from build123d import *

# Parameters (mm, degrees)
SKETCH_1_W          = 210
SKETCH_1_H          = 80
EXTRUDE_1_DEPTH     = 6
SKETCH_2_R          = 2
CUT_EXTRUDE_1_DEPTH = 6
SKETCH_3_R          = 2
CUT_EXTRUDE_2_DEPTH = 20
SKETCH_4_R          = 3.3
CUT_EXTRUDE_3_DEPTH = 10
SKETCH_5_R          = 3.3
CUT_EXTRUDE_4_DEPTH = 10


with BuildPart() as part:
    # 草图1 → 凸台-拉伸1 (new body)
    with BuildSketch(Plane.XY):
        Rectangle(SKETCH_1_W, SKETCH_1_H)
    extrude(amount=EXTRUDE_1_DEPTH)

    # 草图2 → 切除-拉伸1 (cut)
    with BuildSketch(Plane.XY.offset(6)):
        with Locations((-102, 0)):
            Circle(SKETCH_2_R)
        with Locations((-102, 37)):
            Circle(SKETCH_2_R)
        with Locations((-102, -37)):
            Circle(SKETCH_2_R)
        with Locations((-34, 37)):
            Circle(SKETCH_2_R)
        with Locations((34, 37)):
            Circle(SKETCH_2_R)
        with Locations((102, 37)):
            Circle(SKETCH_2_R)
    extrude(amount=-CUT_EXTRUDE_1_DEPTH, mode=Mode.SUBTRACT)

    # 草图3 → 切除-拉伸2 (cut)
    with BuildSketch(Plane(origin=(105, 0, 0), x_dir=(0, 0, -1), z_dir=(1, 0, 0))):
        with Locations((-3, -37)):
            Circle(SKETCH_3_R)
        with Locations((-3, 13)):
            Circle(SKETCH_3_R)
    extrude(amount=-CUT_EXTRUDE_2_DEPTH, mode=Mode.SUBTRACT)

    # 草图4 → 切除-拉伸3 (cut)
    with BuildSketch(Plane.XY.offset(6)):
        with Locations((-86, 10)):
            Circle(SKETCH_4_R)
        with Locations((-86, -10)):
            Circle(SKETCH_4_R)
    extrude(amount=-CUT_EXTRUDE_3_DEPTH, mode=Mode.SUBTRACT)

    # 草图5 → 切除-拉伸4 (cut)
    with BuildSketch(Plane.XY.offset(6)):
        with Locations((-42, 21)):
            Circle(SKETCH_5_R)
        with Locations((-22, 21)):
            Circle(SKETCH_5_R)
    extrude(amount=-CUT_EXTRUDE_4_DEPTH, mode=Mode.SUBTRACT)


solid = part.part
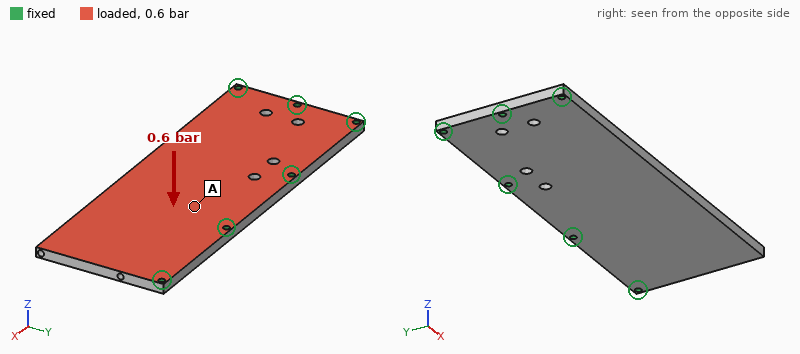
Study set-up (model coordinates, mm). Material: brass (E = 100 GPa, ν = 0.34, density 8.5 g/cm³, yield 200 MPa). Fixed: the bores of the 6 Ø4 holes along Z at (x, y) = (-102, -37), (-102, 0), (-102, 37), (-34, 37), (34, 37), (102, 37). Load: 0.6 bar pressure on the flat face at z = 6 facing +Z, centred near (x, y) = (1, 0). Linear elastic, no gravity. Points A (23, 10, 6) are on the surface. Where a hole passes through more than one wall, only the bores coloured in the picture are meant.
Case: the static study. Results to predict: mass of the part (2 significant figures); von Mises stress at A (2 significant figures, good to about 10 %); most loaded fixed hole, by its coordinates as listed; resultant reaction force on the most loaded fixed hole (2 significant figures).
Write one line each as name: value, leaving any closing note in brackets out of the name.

mass of the part: 840 g
von Mises stress at A: 10 MPa
most loaded fixed hole, by its coordinates as listed: (34, 37)
resultant reaction force on the most loaded fixed hole: 370 N
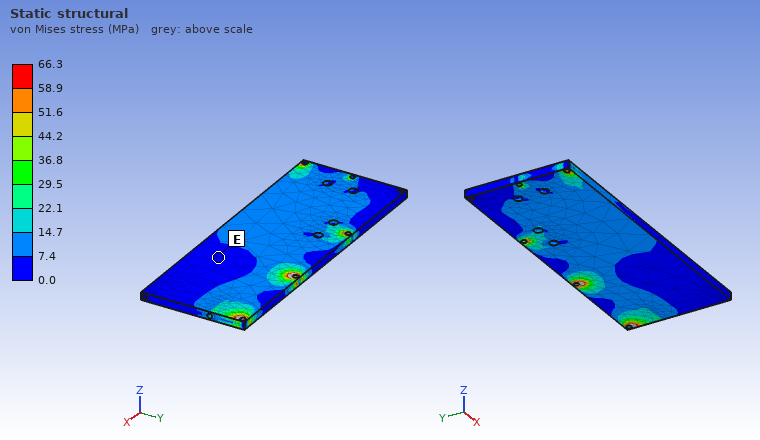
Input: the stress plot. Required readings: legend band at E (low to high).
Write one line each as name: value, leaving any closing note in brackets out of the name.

legend band at E: 0.0 to 7.4 MPa
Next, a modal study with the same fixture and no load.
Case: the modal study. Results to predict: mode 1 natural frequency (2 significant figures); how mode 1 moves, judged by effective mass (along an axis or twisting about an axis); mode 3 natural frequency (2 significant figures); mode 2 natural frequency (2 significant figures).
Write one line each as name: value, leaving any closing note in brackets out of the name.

mode 1 natural frequency: 480 Hz
how mode 1 moves, judged by effective mass: along Z
mode 3 natural frequency: 1800 Hz
mode 2 natural frequency: 960 Hz
